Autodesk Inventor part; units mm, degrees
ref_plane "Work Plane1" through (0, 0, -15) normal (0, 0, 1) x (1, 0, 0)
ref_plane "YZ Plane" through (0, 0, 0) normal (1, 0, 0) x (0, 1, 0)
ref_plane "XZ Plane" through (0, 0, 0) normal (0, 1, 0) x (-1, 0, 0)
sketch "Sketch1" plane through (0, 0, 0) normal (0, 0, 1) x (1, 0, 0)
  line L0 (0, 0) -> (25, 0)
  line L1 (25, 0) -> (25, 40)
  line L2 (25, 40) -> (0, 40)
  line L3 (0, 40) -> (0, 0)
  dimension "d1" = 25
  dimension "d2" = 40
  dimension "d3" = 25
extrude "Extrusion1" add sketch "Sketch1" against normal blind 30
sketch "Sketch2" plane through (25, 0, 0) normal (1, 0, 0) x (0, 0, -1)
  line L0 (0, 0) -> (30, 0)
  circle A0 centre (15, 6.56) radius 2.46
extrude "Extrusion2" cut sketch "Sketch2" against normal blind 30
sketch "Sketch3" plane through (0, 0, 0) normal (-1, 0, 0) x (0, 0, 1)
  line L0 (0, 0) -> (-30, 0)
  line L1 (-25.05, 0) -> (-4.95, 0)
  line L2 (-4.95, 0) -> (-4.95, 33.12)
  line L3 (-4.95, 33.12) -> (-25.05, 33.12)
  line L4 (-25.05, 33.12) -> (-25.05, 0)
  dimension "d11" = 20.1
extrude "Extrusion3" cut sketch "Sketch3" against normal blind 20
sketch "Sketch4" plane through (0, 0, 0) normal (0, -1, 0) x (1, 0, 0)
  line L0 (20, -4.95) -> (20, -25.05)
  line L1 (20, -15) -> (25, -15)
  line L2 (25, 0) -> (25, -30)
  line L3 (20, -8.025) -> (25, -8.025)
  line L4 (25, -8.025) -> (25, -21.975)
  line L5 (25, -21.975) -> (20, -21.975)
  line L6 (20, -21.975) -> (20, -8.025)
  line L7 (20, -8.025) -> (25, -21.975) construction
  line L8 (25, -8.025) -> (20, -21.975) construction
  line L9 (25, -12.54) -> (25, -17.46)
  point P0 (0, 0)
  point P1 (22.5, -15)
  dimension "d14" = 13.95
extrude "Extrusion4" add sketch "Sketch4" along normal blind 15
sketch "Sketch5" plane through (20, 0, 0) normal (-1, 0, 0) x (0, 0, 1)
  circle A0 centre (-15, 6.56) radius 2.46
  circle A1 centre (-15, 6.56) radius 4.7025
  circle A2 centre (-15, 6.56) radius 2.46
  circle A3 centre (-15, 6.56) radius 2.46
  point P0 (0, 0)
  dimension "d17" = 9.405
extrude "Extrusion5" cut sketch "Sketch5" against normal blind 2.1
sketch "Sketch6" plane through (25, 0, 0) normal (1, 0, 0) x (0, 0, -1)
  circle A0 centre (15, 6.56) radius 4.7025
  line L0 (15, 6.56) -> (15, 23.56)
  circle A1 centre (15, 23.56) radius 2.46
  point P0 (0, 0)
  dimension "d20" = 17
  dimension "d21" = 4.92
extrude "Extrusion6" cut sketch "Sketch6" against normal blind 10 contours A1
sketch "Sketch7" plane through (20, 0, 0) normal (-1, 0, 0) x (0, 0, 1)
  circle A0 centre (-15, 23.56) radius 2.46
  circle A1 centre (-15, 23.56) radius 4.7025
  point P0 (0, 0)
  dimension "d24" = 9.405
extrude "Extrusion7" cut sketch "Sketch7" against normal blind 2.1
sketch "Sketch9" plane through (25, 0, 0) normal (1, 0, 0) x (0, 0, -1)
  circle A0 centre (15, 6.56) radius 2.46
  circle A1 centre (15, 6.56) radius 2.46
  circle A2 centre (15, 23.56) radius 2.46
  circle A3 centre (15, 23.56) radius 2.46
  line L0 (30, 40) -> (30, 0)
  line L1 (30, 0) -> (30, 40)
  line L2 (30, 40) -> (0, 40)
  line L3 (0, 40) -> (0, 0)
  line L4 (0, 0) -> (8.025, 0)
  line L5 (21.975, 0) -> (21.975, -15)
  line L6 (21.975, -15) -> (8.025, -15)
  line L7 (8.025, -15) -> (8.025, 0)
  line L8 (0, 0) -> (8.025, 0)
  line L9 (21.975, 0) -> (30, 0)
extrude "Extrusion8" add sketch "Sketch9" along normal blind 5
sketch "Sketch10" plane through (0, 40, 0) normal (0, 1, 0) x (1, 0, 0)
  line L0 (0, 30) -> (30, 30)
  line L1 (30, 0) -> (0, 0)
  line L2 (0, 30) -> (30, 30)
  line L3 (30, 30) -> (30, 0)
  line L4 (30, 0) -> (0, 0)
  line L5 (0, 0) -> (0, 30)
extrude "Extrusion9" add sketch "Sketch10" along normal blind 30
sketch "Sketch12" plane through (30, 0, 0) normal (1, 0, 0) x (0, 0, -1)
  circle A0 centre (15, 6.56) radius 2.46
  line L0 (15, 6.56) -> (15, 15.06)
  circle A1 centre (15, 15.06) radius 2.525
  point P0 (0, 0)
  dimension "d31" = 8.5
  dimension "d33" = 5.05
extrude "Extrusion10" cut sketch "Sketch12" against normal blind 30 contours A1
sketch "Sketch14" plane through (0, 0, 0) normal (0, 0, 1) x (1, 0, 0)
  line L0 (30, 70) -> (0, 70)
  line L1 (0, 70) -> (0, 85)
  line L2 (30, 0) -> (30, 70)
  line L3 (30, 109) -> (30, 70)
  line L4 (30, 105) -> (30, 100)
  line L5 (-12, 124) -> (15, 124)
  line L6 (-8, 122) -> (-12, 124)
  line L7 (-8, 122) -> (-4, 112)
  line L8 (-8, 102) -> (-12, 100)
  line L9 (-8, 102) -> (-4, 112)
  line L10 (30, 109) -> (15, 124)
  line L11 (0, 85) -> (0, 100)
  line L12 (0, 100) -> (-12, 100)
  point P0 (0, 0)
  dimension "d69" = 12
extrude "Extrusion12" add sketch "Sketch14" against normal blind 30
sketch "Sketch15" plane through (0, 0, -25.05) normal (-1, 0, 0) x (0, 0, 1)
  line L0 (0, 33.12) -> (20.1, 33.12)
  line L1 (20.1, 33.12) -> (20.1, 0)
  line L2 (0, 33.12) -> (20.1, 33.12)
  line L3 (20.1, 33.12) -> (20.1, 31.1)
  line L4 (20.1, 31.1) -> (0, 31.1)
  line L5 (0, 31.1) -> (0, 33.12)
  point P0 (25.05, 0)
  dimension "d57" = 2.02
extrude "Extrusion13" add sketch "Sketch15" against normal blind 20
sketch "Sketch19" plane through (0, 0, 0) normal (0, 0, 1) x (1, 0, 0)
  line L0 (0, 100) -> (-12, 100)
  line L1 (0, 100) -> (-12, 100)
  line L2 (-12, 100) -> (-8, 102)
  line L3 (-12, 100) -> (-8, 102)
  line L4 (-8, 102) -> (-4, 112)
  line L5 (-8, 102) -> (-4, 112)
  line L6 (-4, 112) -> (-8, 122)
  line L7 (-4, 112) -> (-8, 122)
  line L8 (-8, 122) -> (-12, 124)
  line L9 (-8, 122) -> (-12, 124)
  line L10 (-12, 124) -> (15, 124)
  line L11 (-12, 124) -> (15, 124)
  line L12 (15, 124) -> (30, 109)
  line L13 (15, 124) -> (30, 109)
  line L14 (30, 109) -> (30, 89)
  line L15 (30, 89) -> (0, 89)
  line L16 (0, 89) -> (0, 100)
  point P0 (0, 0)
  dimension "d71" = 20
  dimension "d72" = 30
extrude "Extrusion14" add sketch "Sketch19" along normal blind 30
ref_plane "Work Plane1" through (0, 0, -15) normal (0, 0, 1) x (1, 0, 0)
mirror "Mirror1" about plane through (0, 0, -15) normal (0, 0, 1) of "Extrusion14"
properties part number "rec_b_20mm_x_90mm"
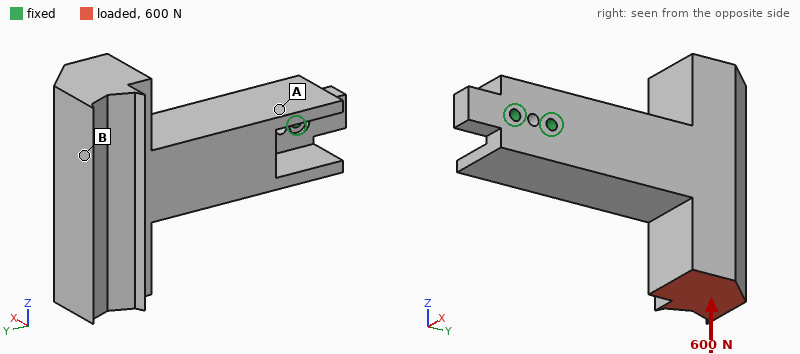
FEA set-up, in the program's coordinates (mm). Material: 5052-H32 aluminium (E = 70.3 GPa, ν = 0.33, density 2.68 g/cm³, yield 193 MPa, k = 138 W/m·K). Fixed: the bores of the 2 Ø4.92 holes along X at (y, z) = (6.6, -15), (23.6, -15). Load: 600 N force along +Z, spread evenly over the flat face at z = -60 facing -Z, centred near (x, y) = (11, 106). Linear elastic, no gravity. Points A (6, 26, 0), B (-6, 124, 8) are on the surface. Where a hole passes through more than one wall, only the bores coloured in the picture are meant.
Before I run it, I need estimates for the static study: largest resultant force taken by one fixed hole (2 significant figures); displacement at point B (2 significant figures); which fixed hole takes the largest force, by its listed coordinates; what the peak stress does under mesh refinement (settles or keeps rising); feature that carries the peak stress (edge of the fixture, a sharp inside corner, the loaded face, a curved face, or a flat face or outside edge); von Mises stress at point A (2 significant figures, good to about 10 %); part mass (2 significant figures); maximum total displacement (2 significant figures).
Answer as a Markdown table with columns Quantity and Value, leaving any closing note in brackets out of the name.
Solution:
| Quantity | Value |
|---|---|
| largest resultant force taken by one fixed hole | 2.7 kN |
| displacement at point B | 0.11 mm |
| which fixed hole takes the largest force, by its listed coordinates | (23.6, -15) |
| what the peak stress does under mesh refinement | keeps rising |
| feature that carries the peak stress | edge of the fixture |
| von Mises stress at point A | 9.9 MPa |
| part mass | 450 g |
| maximum total displacement | 0.12 mm |
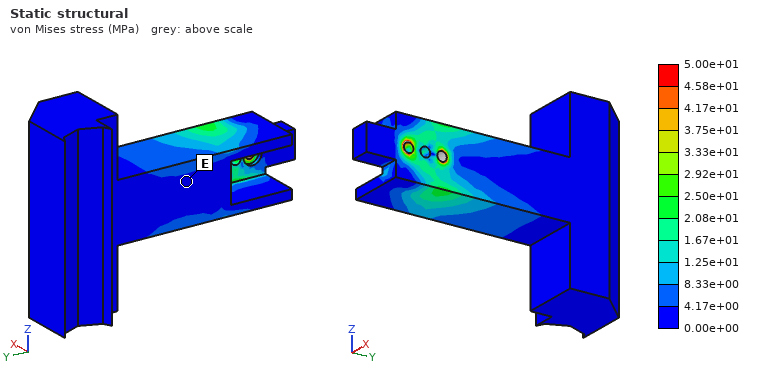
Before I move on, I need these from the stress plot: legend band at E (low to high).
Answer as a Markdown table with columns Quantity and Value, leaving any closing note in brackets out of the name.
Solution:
| Quantity | Value |
|---|---|
| legend band at E | 0.00e+00 to 4.17e+00 MPa |
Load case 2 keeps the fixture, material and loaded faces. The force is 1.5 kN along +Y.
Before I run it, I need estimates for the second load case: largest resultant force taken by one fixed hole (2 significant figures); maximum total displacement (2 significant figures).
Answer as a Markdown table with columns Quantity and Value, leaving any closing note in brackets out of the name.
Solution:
| Quantity | Value |
|---|---|
| largest resultant force taken by one fixed hole | 3.2 kN |
| maximum total displacement | 0.20 mm |
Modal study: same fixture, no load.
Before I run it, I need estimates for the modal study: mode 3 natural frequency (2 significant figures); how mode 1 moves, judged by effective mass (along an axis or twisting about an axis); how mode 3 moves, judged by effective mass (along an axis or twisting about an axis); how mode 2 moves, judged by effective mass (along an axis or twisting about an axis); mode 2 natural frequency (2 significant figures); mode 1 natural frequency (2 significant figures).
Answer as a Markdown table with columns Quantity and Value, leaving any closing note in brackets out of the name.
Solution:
| Quantity | Value |
|---|---|
| mode 3 natural frequency | 1300 Hz |
| how mode 1 moves, judged by effective mass | along X |
| how mode 3 moves, judged by effective mass | twisting about Y |
| how mode 2 moves, judged by effective mass | along Z |
| mode 2 natural frequency | 750 Hz |
| mode 1 natural frequency | 670 Hz |
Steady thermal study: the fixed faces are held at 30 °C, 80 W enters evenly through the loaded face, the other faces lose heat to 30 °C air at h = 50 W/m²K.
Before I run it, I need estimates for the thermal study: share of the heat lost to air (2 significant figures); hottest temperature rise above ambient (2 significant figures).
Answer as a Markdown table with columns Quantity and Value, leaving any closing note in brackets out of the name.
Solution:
| Quantity | Value |
|---|---|
| share of the heat lost to air | 47 % |
| hottest temperature rise above ambient | 57 K |
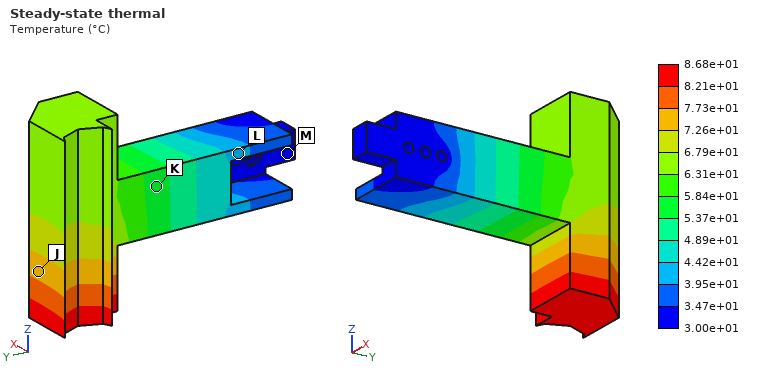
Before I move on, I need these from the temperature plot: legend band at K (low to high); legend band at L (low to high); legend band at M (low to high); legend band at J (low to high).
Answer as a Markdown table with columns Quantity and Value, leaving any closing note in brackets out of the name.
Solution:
| Quantity | Value |
|---|---|
| legend band at K | 5.37e+01 to 5.84e+01 °C |
| legend band at L | 3.95e+01 to 4.42e+01 °C |
| legend band at M | 3.00e+01 to 3.47e+01 °C |
| legend band at J | 7.26e+01 to 7.73e+01 °C |
